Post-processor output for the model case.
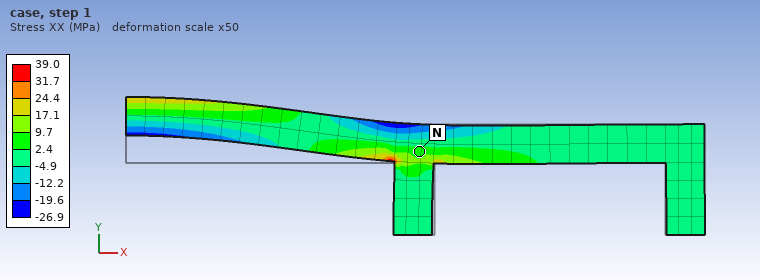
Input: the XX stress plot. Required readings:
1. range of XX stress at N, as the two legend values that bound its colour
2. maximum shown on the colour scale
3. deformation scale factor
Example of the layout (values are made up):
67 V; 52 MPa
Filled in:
2.4 to 9.7 MPa; 39.0 MPa; 50
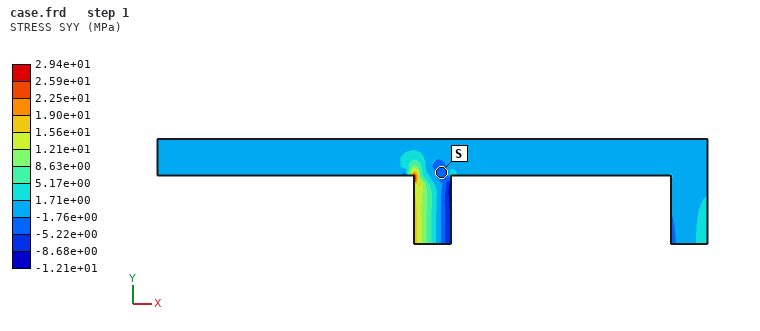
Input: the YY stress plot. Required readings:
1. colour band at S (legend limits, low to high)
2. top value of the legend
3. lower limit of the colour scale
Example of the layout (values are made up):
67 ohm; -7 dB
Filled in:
-5.22e+00 to -1.76e+00 MPa; 2.94e+01 MPa; -1.21e+01 MPa
